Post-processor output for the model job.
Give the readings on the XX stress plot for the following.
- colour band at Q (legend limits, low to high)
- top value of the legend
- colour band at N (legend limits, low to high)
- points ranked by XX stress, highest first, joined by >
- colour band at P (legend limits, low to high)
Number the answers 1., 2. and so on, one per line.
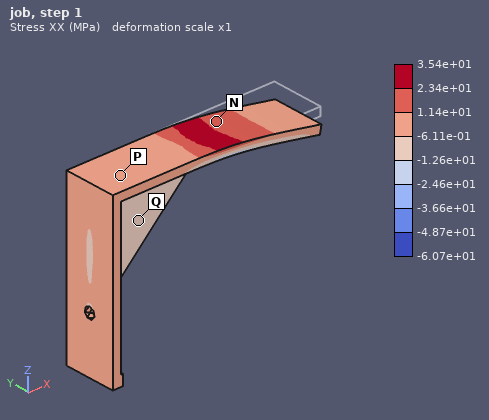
1. -1.26e+01 to -6.11e-01 MPa
2. 3.54e+01 MPa
3. 1.14e+01 to 2.34e+01 MPa
4. N > P > Q
5. -6.11e-01 to 1.14e+01 MPa
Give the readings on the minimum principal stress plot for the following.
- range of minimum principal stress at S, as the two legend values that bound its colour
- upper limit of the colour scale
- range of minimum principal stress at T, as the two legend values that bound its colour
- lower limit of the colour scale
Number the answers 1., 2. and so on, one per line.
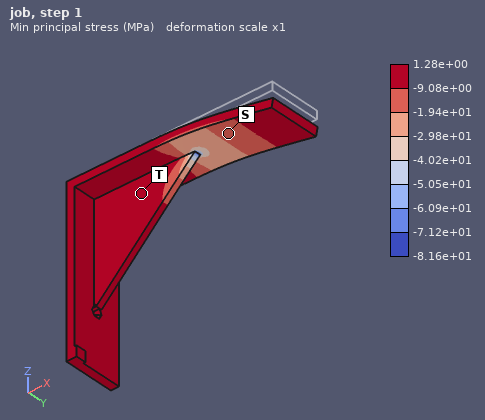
1. -1.94e+01 to -9.08e+00 MPa
2. 1.28e+00 MPa
3. -9.08e+00 to 1.28e+00 MPa
4. -8.16e+01 MPa
